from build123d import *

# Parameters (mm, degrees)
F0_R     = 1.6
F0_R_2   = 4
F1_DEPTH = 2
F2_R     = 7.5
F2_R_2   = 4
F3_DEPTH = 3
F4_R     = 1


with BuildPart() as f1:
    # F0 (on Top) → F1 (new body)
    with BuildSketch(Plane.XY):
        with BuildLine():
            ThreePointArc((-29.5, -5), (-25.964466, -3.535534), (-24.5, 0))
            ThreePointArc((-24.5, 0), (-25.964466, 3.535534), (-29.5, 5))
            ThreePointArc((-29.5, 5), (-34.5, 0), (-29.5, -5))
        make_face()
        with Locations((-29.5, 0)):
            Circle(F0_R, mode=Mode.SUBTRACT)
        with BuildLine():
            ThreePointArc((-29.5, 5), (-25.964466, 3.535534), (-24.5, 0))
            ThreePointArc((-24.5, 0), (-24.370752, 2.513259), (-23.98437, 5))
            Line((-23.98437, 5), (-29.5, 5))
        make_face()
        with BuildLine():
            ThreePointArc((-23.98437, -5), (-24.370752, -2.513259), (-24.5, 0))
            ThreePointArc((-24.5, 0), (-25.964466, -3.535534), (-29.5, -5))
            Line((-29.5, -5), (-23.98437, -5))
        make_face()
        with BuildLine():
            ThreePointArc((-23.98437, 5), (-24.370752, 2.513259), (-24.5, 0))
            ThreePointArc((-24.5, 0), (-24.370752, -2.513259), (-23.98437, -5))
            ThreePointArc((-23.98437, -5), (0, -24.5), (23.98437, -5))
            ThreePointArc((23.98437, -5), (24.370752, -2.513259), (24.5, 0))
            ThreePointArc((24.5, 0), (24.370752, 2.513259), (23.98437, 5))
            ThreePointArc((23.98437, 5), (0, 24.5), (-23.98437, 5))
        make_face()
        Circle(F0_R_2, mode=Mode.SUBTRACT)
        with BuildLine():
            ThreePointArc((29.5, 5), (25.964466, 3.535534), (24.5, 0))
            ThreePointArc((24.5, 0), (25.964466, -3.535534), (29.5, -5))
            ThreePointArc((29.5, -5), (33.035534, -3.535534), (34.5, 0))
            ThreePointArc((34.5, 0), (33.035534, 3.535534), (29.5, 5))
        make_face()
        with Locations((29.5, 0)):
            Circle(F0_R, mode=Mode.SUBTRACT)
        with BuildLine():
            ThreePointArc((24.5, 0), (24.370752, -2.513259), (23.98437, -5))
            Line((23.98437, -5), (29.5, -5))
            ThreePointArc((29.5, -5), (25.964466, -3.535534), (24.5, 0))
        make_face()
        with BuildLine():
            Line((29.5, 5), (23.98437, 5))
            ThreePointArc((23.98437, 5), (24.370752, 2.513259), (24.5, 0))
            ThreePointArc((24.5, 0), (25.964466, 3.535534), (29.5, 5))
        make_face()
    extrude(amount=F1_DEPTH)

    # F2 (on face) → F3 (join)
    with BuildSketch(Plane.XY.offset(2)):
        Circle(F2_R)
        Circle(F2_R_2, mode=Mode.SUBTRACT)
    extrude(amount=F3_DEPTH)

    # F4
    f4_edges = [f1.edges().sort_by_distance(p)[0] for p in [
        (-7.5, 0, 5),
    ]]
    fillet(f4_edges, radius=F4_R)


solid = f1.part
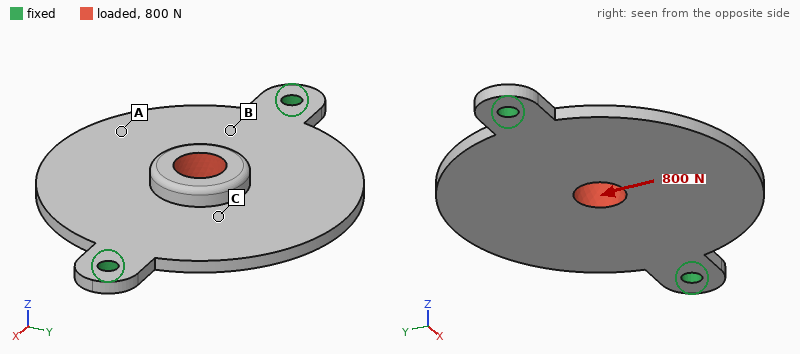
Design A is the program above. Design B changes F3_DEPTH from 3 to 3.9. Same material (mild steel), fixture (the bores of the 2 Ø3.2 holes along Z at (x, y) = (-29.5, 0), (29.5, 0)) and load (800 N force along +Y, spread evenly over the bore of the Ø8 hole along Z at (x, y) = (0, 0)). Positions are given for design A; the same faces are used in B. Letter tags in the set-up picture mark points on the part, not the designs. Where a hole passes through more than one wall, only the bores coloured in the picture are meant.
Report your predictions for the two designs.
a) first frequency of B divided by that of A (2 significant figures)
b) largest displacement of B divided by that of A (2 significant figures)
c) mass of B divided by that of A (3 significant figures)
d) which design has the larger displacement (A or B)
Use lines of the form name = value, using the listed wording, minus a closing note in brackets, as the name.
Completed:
first frequency of B divided by that of A = 1.00
largest displacement of B divided by that of A = 1.3
mass of B divided by that of A = 1.03
which design has the larger displacement = B
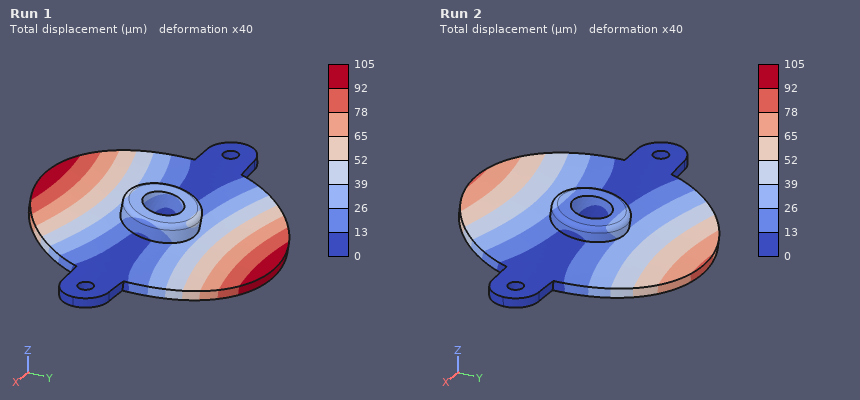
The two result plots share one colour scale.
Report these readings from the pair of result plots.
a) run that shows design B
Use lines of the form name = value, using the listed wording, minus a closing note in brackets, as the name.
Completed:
run that shows design B = Run 1
